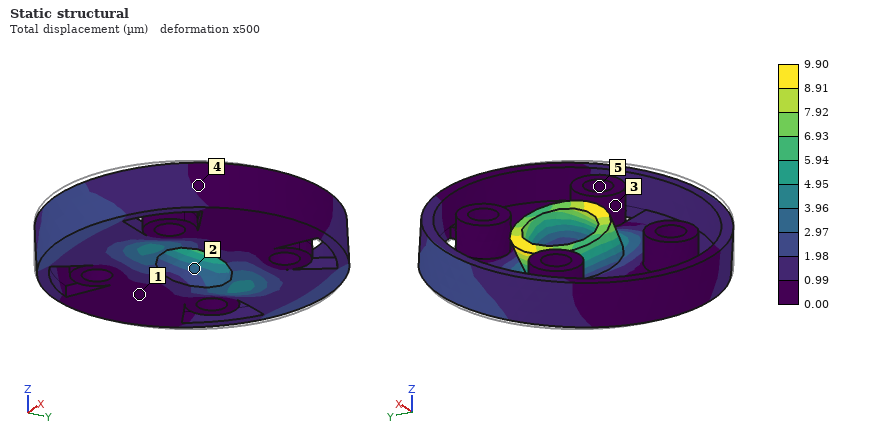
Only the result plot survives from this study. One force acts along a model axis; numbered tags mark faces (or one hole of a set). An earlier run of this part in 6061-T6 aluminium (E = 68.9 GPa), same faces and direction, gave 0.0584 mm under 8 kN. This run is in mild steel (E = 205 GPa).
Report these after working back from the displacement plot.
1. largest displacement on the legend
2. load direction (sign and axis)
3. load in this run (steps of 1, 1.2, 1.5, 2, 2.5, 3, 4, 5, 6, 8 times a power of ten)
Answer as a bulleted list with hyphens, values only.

- 9.90 µm
- +Y
- 4 kN
